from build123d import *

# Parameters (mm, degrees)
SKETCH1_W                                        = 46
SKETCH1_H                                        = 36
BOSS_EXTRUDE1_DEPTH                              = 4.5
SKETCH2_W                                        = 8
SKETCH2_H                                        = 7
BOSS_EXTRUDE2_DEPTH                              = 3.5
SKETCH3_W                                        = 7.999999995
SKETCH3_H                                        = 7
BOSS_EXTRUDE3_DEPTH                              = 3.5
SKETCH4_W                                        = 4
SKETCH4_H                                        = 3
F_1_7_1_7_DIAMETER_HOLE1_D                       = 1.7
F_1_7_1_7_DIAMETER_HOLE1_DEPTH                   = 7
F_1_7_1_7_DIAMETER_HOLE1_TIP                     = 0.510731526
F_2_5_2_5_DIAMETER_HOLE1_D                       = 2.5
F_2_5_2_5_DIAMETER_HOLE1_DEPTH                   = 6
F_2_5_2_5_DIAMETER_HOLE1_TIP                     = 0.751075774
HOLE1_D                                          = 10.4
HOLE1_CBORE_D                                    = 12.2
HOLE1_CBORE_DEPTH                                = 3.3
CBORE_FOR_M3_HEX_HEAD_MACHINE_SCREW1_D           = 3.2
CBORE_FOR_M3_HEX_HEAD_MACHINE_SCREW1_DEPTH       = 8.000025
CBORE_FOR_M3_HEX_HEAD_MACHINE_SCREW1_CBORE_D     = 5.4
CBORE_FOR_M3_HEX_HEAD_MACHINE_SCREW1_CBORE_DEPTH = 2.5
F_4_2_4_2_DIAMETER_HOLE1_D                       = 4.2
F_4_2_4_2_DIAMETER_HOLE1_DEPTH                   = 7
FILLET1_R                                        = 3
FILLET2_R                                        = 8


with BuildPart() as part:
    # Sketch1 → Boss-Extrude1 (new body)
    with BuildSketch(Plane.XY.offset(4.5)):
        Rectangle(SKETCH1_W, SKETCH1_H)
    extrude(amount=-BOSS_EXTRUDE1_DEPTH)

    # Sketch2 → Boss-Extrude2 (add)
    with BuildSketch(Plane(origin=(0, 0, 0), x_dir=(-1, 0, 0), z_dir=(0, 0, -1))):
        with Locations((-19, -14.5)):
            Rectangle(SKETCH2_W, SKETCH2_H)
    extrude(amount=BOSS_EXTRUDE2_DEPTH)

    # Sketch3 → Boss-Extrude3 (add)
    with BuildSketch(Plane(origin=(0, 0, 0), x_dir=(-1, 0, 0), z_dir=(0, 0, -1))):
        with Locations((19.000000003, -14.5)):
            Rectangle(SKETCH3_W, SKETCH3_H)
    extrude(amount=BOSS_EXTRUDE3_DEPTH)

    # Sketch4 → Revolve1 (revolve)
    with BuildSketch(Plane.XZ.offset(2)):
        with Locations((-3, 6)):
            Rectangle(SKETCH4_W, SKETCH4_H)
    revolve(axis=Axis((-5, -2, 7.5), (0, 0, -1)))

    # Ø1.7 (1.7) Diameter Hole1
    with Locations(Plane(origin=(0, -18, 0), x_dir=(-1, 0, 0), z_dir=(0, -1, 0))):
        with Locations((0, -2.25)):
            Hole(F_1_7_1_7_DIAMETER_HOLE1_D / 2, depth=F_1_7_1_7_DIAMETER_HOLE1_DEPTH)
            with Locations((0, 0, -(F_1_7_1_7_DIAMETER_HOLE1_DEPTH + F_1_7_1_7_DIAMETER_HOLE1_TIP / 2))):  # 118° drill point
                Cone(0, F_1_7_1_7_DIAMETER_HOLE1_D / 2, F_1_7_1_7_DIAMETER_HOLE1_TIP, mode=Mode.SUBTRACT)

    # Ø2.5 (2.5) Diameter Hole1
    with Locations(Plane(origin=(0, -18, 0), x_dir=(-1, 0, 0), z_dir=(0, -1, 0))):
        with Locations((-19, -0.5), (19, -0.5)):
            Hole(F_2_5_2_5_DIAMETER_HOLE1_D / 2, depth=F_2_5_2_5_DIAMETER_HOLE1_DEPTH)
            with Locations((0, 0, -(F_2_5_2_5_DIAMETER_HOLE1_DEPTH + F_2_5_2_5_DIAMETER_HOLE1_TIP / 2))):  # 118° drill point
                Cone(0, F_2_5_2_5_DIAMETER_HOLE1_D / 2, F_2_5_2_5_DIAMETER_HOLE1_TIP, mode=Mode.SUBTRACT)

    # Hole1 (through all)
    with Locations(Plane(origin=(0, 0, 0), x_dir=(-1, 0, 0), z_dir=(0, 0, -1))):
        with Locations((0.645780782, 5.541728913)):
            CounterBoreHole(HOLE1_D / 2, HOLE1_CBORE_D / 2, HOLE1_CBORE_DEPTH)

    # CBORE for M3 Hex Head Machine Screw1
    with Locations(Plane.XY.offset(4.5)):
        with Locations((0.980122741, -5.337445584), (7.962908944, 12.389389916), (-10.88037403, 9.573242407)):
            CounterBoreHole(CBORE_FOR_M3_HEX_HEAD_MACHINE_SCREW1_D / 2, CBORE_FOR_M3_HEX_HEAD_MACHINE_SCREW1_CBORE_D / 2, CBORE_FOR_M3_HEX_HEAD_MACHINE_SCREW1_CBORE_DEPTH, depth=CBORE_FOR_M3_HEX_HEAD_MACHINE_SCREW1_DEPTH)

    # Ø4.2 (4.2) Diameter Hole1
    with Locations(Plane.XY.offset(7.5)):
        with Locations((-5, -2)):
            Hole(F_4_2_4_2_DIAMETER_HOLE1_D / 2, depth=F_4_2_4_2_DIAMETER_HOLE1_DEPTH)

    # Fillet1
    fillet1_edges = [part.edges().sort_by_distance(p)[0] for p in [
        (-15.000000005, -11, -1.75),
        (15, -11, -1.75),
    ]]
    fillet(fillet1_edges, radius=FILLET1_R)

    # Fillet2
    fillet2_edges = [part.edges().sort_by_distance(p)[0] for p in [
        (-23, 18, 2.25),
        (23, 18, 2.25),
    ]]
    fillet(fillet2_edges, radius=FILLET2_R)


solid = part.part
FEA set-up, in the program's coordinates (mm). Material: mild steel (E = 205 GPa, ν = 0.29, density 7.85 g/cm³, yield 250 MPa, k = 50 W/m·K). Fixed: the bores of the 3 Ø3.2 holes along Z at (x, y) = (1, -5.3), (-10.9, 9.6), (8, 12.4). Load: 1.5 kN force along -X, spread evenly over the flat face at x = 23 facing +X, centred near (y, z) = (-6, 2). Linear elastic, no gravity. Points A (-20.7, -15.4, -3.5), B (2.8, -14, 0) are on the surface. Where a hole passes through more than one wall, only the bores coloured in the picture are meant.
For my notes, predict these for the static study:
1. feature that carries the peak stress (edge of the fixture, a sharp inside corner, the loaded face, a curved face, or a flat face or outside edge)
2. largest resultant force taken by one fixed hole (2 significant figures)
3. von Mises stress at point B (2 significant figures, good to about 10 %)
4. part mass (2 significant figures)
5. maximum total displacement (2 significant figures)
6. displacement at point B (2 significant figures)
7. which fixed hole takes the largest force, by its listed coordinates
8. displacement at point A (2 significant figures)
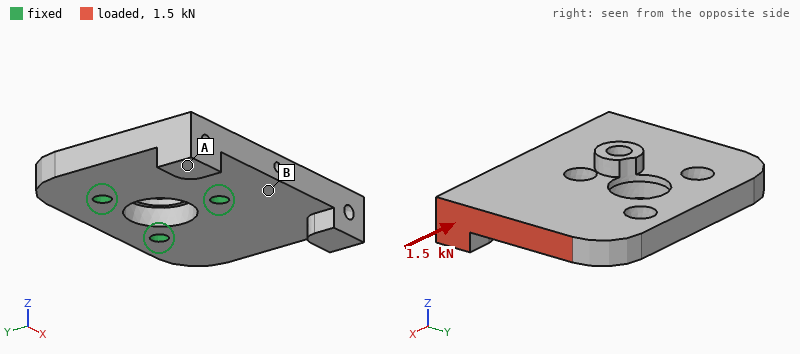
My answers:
edge of the fixture
1.3 kN
17 MPa
55 g
6.9 µm
1.7 µm
(1, -5.3)
2.2 µm
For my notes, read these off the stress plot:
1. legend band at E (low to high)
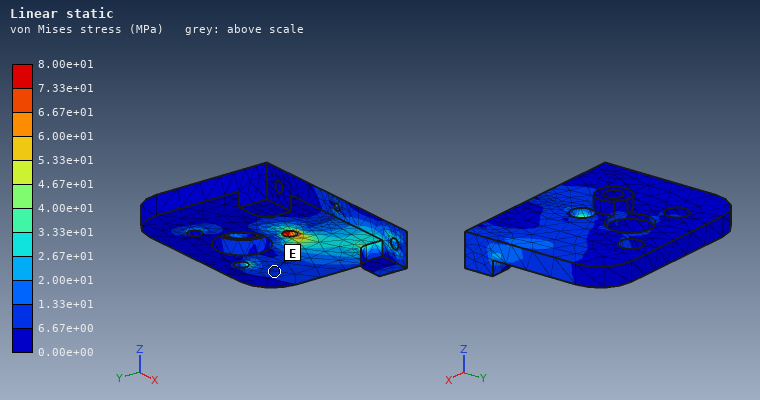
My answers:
6.67e+00 to 1.33e+01 MPa
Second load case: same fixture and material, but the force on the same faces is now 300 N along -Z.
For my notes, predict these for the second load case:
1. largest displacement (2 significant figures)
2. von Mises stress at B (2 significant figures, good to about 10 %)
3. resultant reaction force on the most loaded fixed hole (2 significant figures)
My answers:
42 µm
39 MPa
320 N
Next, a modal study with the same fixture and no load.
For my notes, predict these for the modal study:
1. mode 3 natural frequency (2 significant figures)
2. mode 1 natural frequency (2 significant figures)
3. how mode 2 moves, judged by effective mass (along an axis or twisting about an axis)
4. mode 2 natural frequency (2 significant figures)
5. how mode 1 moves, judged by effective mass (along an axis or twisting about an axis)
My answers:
13 kHz
5100 Hz
along Z
6400 Hz
twisting about Y
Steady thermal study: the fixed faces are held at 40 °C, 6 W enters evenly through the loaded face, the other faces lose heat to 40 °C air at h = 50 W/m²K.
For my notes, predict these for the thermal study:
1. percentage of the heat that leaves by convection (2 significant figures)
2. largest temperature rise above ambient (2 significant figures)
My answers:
18 %
22 K
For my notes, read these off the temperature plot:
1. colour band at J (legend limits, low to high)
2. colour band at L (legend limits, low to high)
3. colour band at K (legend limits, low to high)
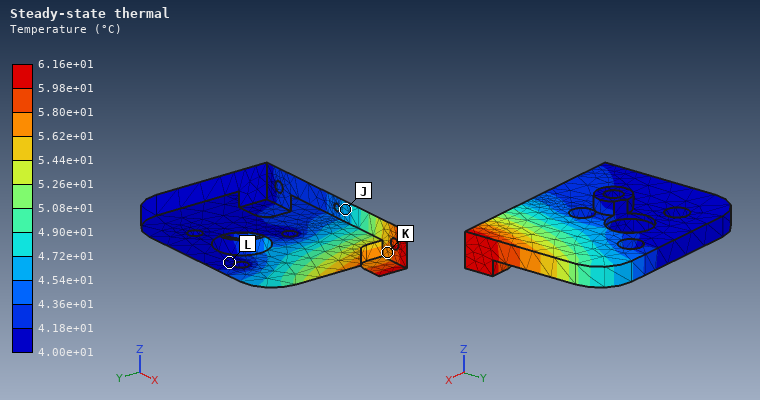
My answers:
4.54e+01 to 4.72e+01 °C
4.00e+01 to 4.18e+01 °C
5.62e+01 to 5.80e+01 °C
